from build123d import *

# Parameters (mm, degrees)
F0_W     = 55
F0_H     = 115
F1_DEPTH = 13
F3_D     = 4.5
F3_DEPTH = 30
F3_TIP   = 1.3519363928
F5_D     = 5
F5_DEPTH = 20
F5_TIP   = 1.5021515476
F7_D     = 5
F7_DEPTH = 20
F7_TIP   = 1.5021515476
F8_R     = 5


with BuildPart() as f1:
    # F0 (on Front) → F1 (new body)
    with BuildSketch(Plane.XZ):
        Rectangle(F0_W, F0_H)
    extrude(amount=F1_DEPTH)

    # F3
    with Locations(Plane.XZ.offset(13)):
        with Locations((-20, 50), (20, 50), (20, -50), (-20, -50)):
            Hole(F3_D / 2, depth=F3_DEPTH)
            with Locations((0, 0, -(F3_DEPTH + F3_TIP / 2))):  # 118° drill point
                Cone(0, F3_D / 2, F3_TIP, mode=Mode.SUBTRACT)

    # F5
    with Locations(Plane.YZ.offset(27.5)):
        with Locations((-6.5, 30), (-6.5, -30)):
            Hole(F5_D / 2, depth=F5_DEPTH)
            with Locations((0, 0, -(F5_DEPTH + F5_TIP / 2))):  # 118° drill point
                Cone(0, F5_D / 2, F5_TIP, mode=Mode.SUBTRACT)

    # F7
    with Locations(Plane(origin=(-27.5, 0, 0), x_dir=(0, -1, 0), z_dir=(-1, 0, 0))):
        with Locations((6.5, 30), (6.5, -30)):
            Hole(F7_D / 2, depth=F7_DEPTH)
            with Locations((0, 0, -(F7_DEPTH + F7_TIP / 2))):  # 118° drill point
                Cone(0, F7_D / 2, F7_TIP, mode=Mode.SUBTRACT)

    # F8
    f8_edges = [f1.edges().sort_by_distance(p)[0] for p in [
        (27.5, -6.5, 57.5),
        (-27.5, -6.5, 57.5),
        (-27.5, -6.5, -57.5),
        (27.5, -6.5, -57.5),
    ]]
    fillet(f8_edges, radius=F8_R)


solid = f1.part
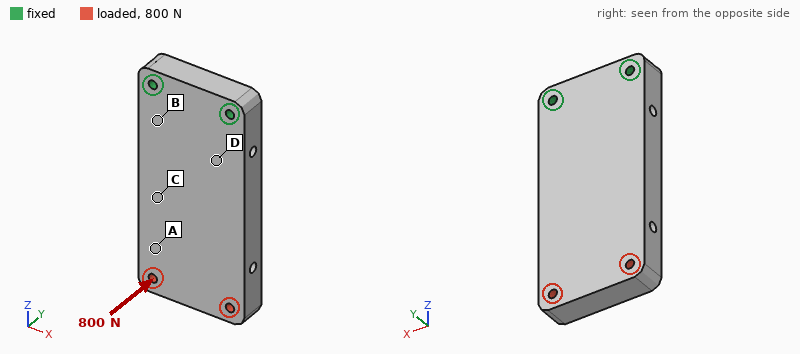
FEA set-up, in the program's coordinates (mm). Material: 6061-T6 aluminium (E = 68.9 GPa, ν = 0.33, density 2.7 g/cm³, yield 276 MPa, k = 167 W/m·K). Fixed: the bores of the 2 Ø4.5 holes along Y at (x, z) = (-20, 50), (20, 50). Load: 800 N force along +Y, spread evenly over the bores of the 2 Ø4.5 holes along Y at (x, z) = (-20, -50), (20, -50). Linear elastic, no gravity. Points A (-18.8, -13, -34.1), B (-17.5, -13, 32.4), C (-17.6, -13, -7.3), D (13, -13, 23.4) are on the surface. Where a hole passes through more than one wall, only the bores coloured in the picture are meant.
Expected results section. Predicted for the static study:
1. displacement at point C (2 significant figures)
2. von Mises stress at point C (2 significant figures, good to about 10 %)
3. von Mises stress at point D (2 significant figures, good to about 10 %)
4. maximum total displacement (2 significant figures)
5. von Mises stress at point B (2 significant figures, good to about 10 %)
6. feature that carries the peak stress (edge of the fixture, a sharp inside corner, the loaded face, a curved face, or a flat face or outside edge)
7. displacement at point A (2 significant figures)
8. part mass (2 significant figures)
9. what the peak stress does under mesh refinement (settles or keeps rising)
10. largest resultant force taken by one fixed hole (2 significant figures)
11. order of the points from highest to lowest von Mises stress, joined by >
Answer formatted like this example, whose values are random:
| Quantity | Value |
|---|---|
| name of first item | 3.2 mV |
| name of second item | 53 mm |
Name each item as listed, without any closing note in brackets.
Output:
| Quantity | Value |
|---|---|
| displacement at point C | 0.19 mm |
| von Mises stress at point C | 22 MPa |
| von Mises stress at point D | 37 MPa |
| maximum total displacement | 0.50 mm |
| von Mises stress at point B | 47 MPa |
| feature that carries the peak stress | edge of the fixture |
| displacement at point A | 0.35 mm |
| part mass | 210 g |
| what the peak stress does under mesh refinement | keeps rising |
| largest resultant force taken by one fixed hole | 400 N |
| order of the points from highest to lowest von Mises stress, joined by > | B > D > C > A |
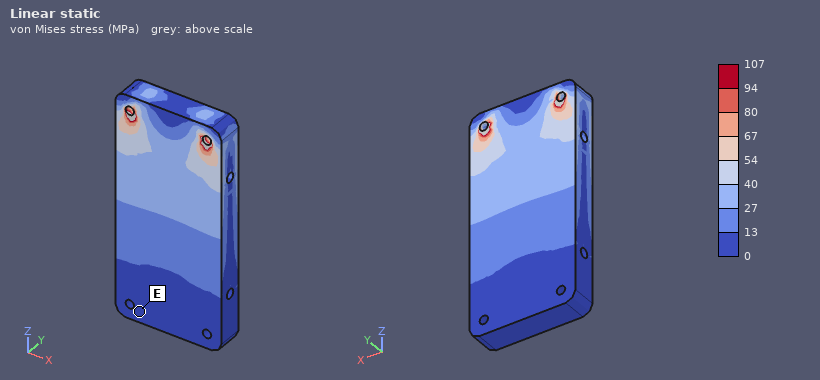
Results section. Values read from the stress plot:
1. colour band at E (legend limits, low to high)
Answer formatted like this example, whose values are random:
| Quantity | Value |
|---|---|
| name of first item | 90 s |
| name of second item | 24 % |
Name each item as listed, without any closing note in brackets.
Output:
| Quantity | Value |
|---|---|
| colour band at E | 0 to 13 MPa |
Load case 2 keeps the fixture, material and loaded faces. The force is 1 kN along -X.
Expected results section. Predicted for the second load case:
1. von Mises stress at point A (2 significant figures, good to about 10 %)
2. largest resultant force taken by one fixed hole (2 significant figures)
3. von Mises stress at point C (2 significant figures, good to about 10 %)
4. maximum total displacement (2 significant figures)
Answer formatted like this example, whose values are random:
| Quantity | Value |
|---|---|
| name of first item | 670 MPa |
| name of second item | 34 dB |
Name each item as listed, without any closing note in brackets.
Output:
| Quantity | Value |
|---|---|
| von Mises stress at point A | 3.2 MPa |
| largest resultant force taken by one fixed hole | 2.5 kN |
| von Mises stress at point C | 4.7 MPa |
| maximum total displacement | 43 µm |
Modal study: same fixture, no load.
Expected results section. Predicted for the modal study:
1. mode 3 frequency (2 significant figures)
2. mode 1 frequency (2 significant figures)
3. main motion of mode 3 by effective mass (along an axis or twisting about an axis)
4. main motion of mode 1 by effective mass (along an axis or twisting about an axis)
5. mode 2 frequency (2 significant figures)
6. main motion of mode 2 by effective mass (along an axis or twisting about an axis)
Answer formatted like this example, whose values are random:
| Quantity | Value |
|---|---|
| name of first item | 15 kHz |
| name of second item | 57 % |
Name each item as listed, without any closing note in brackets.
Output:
| Quantity | Value |
|---|---|
| mode 3 frequency | 3500 Hz |
| mode 1 frequency | 850 Hz |
| main motion of mode 3 by effective mass | twisting about Z |
| main motion of mode 1 by effective mass | along Y |
| mode 2 frequency | 3100 Hz |
| main motion of mode 2 by effective mass | along X |
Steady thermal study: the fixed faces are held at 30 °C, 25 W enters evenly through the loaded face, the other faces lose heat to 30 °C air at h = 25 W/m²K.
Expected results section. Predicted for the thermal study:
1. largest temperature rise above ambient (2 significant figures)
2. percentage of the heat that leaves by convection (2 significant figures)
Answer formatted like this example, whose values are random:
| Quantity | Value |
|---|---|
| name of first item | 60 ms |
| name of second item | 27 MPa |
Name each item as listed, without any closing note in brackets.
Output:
| Quantity | Value |
|---|---|
| largest temperature rise above ambient | 22 K |
| percentage of the heat that leaves by convection | 18 % |
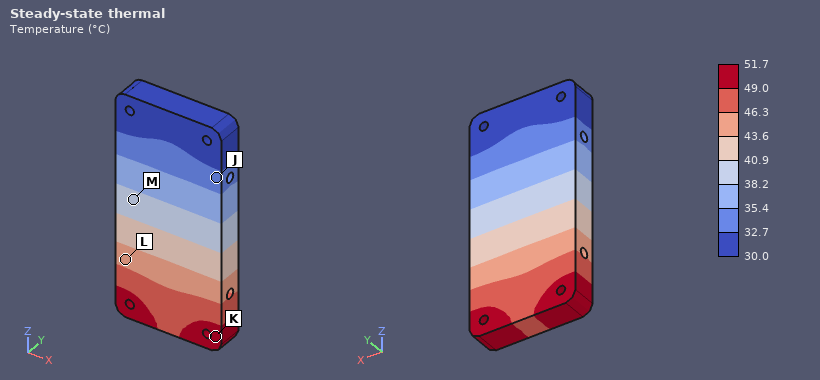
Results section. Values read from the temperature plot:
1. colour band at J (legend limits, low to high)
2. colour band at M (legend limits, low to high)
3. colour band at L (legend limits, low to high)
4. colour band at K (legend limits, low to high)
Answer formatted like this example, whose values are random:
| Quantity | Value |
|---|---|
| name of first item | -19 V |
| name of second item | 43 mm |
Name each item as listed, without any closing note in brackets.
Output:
| Quantity | Value |
|---|---|
| colour band at J | 32.7 to 35.4 °C |
| colour band at M | 38.2 to 40.9 °C |
| colour band at L | 43.6 to 46.3 °C |
| colour band at K | 49.0 to 51.7 °C |
